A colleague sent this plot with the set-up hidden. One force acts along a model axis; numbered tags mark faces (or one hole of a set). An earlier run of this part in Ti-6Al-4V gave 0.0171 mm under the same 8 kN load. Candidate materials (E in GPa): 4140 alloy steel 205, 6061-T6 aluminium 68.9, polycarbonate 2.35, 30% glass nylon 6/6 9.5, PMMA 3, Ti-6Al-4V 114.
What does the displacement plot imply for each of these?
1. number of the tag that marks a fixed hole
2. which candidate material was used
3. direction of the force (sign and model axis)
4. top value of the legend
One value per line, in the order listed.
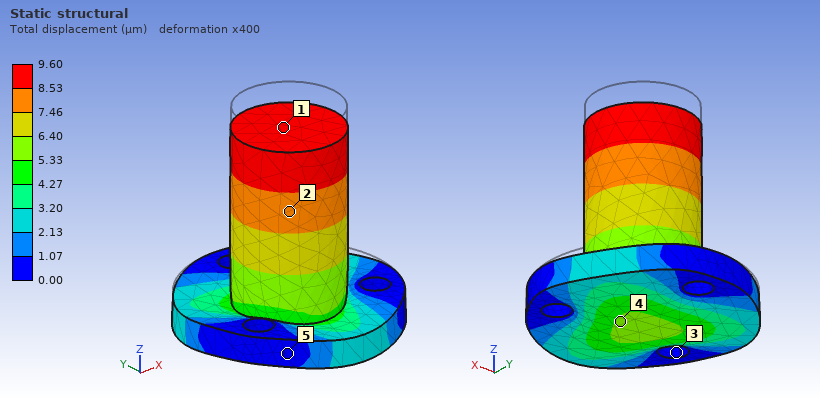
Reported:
3
4140 alloy steel
-Z
9.60 µm
